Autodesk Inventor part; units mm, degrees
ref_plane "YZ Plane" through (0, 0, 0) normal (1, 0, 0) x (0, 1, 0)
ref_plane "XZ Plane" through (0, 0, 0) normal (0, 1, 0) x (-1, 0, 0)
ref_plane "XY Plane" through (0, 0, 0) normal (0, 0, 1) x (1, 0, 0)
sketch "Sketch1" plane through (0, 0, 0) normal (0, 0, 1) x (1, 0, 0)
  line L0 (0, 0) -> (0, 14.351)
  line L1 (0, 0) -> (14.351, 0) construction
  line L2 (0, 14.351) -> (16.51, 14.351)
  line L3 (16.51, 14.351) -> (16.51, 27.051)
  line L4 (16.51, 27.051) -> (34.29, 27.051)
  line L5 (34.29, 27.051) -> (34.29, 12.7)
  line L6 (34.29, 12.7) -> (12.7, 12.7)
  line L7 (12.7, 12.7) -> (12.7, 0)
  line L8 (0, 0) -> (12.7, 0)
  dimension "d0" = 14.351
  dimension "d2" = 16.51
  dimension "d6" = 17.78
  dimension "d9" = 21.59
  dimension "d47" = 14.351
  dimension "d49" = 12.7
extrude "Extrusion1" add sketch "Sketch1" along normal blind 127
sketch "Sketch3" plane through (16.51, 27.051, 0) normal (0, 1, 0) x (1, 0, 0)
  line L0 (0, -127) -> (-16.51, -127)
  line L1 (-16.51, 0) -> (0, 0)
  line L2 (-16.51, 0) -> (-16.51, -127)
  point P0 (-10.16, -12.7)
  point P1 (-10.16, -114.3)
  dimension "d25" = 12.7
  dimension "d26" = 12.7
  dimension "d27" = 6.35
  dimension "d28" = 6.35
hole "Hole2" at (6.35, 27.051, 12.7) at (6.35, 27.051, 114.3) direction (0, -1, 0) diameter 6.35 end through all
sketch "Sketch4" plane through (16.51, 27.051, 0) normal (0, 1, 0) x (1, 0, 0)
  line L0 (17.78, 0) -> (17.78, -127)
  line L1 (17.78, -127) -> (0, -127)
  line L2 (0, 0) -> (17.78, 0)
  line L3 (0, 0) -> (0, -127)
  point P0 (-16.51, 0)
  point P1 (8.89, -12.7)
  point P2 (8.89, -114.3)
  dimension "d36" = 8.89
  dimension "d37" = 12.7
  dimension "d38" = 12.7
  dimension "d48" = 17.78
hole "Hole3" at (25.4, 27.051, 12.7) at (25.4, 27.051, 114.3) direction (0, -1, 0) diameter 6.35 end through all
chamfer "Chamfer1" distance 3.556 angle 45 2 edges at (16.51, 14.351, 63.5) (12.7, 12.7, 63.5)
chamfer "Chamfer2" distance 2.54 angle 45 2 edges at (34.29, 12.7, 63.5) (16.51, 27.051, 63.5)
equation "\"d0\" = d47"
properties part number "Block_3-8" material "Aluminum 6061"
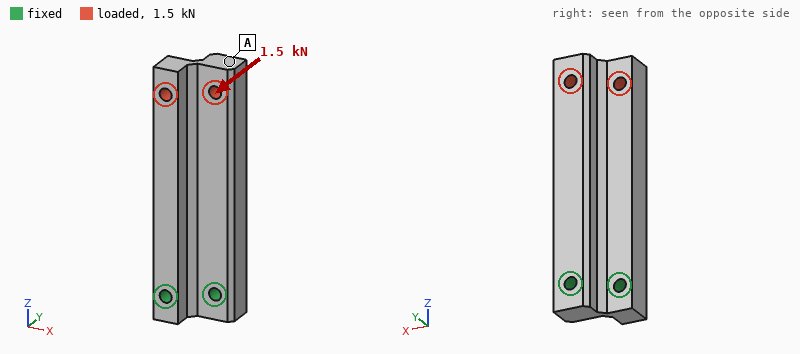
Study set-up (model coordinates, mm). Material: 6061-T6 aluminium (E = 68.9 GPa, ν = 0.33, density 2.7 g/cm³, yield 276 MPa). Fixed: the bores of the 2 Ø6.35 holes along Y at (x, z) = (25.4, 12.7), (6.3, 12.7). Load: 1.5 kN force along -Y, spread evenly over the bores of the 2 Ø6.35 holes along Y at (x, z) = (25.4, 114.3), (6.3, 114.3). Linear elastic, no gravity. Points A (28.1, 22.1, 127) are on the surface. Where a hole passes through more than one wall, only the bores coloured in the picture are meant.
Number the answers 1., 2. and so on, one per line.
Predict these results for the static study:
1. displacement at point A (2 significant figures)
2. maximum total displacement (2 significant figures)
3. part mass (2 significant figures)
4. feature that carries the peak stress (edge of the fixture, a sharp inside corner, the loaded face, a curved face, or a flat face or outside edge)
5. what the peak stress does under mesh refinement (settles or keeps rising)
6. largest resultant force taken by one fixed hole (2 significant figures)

1. 1.0 mm
2. 1.0 mm
3. 150 g
4. edge of the fixture
5. keeps rising
6. 2.5 kN
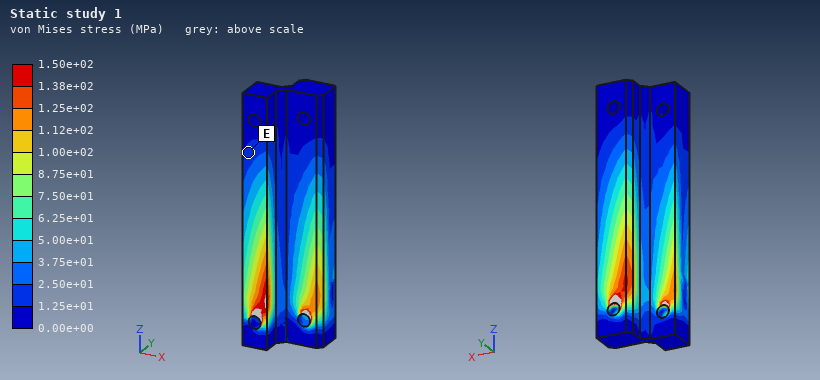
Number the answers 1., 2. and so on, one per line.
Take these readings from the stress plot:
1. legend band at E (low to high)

1. 1.25e+01 to 2.50e+01 MPa
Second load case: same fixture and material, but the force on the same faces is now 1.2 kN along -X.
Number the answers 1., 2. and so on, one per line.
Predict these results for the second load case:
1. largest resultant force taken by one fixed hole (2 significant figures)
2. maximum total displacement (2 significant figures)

1. 4.2 kN
2. 0.57 mm
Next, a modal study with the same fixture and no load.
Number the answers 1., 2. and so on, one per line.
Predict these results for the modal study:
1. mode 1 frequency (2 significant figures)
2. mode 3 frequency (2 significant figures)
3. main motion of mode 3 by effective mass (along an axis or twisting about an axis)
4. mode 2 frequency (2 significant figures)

1. 890 Hz
2. 3400 Hz
3. twisting about Z
4. 2300 Hz
